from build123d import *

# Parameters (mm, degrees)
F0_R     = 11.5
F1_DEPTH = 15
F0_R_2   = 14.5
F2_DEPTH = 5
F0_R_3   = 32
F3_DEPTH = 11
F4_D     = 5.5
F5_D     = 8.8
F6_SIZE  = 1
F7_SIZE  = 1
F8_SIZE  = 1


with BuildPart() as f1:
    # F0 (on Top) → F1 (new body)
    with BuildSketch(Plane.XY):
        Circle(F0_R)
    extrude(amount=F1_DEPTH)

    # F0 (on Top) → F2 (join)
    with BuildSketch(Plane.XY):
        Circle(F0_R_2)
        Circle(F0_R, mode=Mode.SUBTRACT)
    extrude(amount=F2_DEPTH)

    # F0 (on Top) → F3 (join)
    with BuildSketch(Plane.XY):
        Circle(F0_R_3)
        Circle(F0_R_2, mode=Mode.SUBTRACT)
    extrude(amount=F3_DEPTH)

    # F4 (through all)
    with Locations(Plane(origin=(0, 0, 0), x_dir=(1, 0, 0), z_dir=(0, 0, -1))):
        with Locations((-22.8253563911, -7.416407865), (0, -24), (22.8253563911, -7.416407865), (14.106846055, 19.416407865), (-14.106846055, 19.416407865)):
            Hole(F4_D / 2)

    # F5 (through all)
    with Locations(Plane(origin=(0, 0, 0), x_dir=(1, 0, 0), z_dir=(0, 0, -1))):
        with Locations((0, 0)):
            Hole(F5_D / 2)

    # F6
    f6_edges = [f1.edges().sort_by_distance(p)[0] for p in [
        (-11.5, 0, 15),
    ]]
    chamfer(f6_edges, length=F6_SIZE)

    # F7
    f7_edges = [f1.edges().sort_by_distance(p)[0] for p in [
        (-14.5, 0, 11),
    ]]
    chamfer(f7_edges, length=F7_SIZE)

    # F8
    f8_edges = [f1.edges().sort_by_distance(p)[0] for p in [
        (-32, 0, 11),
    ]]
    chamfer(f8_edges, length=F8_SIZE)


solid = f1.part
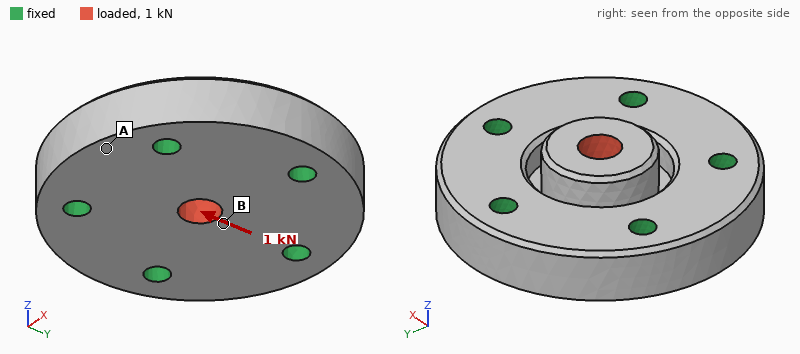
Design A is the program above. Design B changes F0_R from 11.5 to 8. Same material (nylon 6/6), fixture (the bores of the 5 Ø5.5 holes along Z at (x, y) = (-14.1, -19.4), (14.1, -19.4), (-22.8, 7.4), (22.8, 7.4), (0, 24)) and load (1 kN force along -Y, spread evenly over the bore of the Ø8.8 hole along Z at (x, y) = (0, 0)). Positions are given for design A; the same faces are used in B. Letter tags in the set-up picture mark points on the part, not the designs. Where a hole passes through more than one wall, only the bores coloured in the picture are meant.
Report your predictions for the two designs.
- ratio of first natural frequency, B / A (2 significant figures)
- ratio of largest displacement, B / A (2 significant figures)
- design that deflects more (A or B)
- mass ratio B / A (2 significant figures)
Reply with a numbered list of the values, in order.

1. 1.0
2. 2.4
3. B
4. 0.94
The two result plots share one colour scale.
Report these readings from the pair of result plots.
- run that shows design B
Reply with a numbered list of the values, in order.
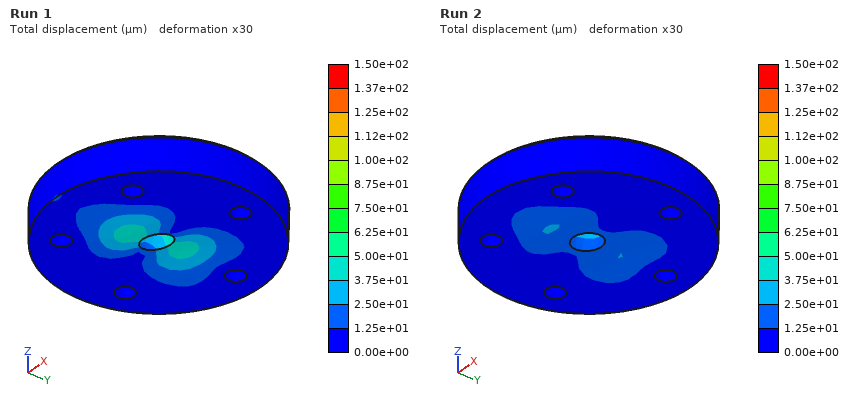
1. Run 1
